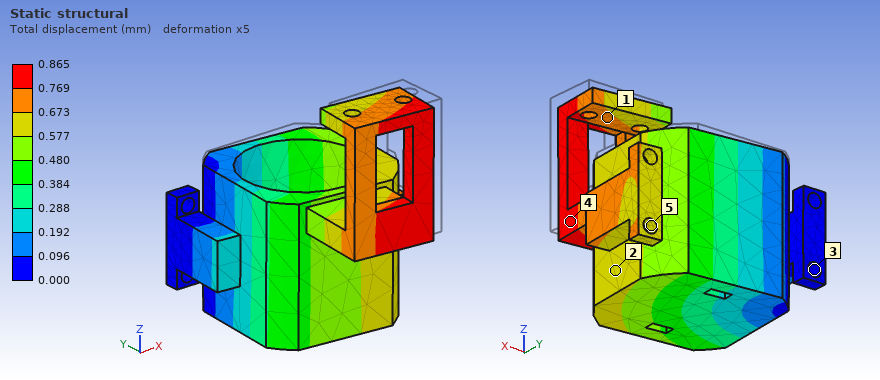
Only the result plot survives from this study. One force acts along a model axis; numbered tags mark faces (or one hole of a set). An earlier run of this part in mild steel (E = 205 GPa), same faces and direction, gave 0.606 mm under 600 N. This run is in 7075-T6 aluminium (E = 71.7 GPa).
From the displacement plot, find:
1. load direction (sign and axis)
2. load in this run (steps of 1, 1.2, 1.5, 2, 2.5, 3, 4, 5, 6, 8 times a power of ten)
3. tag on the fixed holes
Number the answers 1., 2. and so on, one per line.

1. -Y
2. 300 N
3. 3
